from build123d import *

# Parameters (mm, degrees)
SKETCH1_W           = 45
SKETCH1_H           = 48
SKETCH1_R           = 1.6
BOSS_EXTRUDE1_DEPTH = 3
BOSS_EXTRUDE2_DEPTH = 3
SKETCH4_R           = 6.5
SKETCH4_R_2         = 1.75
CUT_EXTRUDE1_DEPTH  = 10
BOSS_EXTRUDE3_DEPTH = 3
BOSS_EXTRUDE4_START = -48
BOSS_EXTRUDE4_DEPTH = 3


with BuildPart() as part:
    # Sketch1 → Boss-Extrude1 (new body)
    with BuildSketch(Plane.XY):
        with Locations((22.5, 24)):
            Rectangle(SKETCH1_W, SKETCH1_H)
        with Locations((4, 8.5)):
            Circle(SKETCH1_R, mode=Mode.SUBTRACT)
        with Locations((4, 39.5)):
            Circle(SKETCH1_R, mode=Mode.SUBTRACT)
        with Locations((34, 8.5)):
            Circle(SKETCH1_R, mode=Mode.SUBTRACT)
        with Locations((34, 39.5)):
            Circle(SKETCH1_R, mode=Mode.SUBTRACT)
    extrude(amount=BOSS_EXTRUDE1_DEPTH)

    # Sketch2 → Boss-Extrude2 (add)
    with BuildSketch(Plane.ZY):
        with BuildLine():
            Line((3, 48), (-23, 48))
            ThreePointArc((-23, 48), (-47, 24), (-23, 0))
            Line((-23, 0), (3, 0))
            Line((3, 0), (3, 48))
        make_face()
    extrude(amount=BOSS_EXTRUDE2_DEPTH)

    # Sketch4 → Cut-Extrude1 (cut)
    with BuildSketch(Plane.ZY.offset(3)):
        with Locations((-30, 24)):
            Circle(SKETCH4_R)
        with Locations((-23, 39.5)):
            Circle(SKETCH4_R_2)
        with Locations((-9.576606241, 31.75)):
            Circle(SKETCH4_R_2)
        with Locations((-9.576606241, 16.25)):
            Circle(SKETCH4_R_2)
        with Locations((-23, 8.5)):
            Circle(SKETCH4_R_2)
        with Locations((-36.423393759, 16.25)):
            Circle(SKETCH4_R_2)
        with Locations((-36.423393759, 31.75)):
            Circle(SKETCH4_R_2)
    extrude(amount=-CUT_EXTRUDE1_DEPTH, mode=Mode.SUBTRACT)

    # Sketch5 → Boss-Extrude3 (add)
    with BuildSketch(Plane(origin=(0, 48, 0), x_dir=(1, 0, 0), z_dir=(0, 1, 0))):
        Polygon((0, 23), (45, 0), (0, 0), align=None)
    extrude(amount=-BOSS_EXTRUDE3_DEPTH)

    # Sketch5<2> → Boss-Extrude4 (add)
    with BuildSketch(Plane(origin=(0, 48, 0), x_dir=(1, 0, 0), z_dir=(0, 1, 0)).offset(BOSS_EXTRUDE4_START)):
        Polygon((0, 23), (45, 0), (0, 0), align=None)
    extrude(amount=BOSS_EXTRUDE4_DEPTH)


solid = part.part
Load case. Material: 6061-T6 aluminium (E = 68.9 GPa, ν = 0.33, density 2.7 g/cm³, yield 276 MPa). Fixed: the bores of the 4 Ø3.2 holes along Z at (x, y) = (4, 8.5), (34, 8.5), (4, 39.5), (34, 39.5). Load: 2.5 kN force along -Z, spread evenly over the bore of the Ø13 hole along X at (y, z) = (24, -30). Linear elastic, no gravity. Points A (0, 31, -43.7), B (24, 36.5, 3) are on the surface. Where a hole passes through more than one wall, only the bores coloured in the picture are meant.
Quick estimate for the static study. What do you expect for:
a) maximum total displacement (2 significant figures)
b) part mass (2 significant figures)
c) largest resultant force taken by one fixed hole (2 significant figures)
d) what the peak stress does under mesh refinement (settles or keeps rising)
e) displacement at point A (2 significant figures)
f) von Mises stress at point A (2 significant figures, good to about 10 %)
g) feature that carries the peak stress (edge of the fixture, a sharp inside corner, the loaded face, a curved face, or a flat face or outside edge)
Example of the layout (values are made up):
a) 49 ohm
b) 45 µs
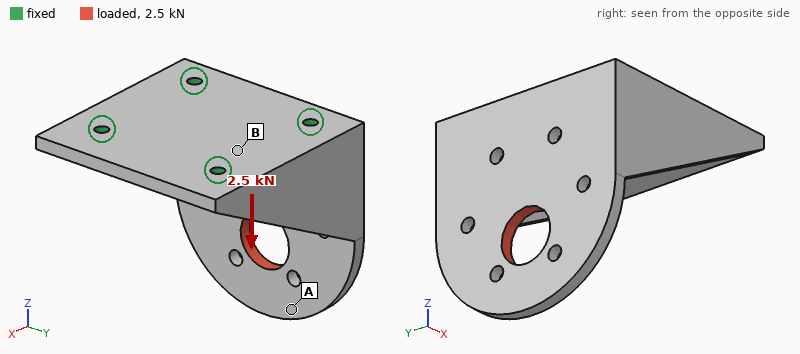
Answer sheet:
a) 67 µm
b) 42 g
c) 1.4 kN
d) keeps rising
e) 61 µm
f) 23 MPa
g) edge of the fixture
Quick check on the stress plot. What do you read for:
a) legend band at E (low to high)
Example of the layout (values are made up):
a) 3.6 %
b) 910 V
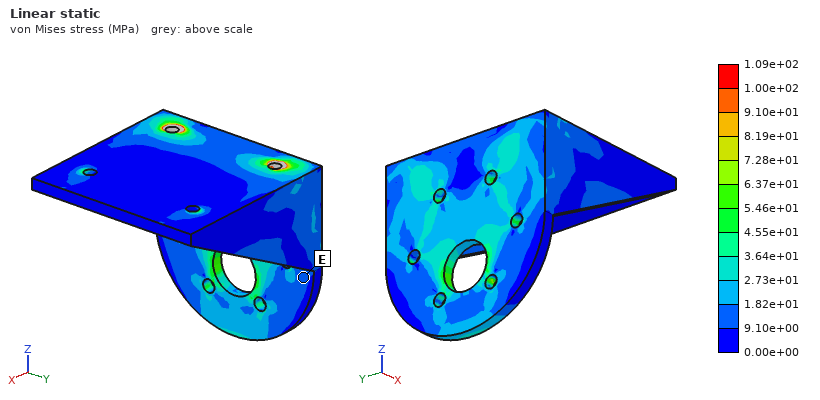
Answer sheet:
a) 9.10e+00 to 1.82e+01 MPa
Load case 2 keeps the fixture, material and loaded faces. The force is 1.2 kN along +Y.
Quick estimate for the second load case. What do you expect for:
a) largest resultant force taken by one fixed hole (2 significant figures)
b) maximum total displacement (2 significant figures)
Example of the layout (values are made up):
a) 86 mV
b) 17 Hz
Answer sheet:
a) 1.3 kN
b) 75 µm
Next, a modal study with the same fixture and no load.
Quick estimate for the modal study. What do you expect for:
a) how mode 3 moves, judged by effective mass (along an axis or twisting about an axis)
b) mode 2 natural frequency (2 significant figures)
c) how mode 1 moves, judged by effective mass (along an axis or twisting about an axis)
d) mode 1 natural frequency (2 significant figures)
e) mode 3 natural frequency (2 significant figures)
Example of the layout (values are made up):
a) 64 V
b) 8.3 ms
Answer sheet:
a) along Y
b) 6100 Hz
c) along X
d) 2500 Hz
e) 7500 Hz
